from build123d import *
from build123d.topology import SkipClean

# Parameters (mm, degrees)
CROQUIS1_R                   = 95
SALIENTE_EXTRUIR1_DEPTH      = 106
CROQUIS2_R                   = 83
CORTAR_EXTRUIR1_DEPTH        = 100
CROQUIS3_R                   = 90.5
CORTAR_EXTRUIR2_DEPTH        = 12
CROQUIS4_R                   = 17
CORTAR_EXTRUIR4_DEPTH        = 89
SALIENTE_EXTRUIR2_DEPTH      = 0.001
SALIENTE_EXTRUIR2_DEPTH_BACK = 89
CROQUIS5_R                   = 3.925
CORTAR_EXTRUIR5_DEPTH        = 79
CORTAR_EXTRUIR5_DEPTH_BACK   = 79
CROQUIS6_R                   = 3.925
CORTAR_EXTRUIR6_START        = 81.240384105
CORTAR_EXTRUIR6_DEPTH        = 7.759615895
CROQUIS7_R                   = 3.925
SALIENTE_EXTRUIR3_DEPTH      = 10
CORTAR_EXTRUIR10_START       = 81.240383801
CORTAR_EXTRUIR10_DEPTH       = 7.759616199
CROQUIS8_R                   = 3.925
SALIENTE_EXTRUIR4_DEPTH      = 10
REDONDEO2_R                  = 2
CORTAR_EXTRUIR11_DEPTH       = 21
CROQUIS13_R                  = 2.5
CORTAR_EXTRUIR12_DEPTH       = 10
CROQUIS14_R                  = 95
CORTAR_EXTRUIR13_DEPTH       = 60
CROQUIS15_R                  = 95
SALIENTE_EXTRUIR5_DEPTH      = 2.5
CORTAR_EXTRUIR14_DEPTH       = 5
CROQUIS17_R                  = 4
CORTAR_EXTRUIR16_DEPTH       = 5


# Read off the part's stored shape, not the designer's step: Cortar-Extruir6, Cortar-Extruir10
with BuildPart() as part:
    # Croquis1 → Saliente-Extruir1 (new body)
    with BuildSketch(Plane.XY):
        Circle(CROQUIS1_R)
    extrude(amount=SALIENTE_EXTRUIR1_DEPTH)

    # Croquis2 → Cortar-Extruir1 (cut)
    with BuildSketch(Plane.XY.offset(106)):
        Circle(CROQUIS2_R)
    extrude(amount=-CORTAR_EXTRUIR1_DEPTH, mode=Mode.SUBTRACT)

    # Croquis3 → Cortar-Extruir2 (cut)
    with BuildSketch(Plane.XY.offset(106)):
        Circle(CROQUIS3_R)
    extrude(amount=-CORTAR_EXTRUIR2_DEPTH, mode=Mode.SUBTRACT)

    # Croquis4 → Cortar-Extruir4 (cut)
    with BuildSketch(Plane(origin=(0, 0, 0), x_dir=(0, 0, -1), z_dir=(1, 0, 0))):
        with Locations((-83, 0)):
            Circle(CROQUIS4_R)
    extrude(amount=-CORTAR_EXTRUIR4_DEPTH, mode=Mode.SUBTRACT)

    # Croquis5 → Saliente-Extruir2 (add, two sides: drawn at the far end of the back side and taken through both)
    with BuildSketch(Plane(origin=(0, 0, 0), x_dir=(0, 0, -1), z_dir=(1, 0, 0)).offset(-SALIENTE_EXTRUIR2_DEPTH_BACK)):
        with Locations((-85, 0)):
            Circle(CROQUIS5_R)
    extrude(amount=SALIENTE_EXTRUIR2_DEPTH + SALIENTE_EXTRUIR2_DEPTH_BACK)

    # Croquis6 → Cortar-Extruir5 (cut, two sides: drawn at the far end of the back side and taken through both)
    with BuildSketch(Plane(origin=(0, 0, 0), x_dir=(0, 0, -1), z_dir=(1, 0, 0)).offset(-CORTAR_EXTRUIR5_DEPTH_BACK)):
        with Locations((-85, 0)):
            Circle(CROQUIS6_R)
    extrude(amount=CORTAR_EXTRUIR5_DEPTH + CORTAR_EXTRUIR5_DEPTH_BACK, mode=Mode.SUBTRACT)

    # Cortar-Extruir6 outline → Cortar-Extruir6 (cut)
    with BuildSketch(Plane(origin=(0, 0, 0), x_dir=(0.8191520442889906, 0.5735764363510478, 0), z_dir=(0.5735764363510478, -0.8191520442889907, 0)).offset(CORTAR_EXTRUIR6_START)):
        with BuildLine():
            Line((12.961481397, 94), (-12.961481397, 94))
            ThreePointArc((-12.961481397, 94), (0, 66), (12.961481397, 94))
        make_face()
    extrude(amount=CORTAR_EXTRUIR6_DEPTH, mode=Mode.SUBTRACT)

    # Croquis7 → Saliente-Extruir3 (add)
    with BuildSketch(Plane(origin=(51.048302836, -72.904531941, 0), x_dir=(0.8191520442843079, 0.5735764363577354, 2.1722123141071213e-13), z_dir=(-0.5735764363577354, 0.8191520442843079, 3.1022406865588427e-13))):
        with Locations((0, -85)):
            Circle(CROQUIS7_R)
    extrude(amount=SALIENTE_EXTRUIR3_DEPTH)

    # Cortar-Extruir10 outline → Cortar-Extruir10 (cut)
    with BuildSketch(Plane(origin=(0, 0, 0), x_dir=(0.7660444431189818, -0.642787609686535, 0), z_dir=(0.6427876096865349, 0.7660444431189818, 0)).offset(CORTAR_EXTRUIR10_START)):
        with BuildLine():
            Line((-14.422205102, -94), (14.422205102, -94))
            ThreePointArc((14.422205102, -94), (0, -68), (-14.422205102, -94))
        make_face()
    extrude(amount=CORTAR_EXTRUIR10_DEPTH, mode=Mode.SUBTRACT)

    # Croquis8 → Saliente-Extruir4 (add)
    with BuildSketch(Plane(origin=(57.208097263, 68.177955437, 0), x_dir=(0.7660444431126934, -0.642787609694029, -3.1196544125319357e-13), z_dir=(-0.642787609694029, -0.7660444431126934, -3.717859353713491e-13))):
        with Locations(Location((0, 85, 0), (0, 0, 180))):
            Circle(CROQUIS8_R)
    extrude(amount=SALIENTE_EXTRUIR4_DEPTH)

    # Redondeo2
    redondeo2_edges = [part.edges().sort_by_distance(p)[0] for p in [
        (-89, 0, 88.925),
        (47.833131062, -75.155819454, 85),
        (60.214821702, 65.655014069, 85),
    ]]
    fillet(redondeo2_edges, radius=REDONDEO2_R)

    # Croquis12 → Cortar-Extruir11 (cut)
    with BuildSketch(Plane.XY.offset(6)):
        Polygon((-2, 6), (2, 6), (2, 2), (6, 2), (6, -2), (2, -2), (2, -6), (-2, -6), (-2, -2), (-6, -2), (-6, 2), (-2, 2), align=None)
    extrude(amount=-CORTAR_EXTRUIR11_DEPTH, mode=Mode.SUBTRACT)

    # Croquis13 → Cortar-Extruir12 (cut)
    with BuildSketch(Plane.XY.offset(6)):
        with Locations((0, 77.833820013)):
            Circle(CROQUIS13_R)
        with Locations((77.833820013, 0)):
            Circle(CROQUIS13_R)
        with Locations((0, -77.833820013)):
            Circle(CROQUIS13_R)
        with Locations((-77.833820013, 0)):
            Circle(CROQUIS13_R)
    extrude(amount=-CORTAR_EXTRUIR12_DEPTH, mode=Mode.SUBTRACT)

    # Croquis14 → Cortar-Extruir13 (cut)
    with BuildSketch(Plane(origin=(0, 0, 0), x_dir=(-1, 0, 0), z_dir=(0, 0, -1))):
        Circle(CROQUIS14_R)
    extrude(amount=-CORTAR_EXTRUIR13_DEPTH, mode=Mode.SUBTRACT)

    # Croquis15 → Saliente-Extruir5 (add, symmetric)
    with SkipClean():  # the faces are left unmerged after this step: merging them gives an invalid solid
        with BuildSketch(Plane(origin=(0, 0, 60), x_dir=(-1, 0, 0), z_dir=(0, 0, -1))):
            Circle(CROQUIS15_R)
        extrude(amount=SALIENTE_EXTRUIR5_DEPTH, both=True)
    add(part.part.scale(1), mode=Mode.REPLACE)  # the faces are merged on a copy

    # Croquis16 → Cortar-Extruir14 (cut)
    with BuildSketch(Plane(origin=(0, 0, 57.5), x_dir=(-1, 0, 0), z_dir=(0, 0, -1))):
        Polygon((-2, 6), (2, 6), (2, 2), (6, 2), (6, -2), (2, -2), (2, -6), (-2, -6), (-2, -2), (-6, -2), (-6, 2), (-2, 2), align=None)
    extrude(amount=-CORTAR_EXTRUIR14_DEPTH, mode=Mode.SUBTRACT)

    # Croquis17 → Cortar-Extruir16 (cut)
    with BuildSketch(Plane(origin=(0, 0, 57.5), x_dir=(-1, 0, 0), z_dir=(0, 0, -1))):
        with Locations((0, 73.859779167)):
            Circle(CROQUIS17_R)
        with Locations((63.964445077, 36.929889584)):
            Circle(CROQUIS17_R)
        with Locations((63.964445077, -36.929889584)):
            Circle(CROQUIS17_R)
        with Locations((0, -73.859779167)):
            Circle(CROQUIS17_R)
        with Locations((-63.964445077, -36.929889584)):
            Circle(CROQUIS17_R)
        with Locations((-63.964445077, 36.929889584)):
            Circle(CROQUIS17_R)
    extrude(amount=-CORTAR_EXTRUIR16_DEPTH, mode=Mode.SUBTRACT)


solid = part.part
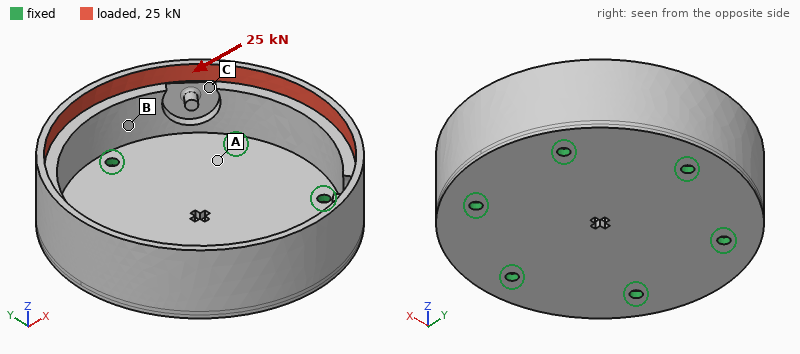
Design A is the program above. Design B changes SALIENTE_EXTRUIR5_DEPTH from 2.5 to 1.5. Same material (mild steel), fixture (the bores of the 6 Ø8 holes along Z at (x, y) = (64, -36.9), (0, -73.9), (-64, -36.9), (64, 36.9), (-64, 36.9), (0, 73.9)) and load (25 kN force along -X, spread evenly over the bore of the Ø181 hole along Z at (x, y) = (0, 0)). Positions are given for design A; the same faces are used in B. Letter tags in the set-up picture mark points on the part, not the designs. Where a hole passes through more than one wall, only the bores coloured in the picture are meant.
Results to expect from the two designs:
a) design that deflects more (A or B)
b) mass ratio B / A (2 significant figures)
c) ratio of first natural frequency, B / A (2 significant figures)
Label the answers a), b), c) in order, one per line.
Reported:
a) B
b) 0.87
c) 0.62
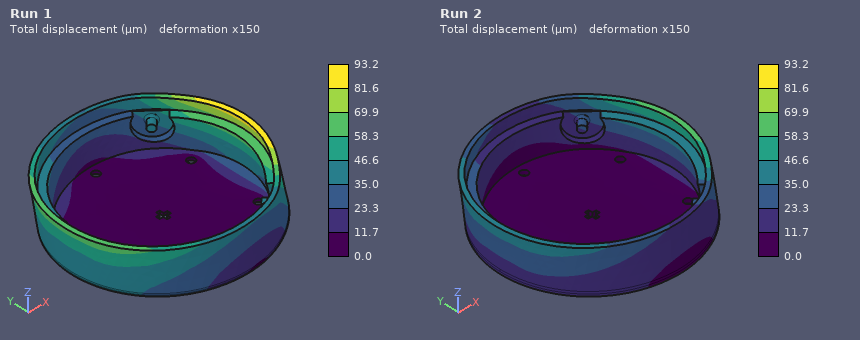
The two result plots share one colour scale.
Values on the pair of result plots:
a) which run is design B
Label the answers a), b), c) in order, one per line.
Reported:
a) Run 1
